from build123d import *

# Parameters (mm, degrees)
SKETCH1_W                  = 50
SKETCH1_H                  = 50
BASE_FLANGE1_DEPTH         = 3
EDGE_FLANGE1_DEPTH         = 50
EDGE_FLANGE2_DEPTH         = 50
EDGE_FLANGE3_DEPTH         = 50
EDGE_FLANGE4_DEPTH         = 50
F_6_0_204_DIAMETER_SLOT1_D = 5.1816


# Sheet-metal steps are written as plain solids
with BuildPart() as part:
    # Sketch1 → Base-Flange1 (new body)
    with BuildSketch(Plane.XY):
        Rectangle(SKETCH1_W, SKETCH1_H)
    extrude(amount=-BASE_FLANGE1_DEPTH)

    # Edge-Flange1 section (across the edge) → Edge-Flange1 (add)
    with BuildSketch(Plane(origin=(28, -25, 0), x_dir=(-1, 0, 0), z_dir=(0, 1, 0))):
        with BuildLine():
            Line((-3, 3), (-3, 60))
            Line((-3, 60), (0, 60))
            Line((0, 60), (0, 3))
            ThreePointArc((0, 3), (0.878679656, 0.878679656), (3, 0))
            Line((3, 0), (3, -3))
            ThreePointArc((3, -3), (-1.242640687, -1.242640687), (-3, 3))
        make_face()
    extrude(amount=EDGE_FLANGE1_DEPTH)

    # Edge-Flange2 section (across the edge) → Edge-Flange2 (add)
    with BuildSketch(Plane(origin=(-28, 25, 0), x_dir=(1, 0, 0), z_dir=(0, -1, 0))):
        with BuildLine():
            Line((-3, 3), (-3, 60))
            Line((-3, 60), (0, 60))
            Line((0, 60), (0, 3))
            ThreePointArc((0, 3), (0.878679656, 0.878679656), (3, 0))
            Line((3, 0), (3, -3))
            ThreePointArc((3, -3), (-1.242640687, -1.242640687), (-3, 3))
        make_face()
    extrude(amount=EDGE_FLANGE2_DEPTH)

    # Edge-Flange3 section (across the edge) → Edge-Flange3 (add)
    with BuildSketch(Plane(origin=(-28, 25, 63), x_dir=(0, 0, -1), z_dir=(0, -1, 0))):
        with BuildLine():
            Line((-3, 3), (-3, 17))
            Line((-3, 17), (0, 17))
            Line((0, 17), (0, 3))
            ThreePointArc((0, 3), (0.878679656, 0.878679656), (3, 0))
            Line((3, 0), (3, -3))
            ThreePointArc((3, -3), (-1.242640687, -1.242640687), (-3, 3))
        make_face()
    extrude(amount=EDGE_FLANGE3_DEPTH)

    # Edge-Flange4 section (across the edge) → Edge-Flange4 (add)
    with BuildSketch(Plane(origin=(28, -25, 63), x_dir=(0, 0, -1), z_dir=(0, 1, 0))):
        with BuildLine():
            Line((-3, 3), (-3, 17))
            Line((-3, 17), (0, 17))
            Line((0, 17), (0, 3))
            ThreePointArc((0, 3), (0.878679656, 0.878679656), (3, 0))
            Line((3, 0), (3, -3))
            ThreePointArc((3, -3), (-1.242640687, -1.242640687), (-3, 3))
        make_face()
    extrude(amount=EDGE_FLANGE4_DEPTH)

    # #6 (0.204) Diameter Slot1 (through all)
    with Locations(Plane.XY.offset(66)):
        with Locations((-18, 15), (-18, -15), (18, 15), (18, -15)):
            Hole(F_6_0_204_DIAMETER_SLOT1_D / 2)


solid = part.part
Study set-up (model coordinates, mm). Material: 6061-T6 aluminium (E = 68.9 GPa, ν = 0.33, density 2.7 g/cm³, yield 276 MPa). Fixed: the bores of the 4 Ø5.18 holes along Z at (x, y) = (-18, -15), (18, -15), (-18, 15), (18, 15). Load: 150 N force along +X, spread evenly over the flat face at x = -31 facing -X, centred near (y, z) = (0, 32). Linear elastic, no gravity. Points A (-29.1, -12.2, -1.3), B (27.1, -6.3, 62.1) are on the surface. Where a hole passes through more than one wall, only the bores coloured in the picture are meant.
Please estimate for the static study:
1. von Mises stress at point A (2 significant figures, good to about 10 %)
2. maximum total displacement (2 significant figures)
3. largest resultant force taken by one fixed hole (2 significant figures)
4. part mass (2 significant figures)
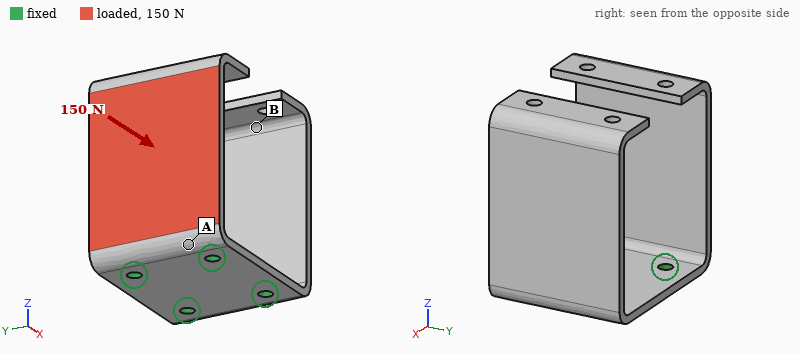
46 MPa
1.0 mm
67 N
88 g
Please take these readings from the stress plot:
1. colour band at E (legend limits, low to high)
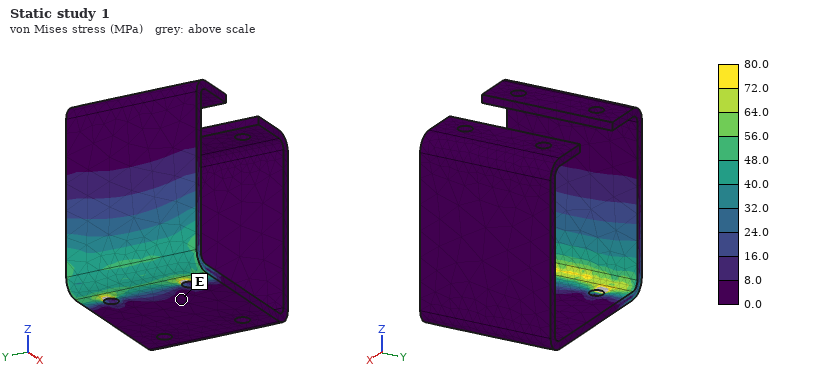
0.0 to 8.0 MPa
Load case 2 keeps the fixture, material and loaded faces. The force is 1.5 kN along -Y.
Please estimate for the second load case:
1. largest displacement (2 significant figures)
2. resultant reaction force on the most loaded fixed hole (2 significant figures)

0.63 mm
1.8 kN
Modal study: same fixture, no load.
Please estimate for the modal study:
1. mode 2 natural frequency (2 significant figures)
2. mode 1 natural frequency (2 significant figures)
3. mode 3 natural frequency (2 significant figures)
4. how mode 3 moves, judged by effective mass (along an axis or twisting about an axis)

340 Hz
340 Hz
1000 Hz
along Y
